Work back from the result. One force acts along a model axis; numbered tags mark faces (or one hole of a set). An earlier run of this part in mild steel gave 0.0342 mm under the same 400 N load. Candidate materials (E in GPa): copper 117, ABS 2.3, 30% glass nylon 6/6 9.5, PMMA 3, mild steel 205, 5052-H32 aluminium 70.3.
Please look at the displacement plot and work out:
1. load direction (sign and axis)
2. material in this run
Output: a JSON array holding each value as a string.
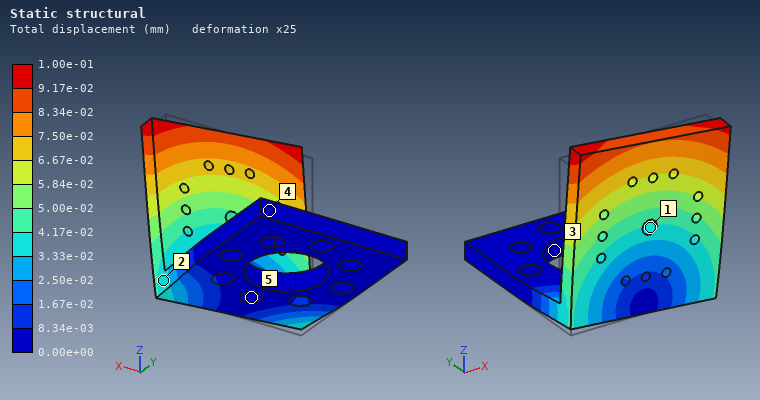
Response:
["+X", "5052-H32 aluminium"]
